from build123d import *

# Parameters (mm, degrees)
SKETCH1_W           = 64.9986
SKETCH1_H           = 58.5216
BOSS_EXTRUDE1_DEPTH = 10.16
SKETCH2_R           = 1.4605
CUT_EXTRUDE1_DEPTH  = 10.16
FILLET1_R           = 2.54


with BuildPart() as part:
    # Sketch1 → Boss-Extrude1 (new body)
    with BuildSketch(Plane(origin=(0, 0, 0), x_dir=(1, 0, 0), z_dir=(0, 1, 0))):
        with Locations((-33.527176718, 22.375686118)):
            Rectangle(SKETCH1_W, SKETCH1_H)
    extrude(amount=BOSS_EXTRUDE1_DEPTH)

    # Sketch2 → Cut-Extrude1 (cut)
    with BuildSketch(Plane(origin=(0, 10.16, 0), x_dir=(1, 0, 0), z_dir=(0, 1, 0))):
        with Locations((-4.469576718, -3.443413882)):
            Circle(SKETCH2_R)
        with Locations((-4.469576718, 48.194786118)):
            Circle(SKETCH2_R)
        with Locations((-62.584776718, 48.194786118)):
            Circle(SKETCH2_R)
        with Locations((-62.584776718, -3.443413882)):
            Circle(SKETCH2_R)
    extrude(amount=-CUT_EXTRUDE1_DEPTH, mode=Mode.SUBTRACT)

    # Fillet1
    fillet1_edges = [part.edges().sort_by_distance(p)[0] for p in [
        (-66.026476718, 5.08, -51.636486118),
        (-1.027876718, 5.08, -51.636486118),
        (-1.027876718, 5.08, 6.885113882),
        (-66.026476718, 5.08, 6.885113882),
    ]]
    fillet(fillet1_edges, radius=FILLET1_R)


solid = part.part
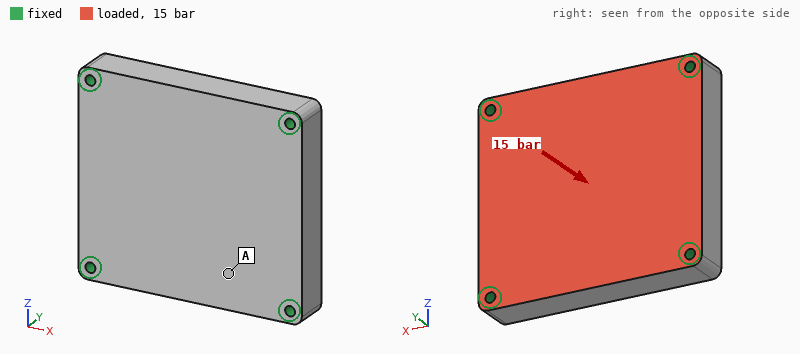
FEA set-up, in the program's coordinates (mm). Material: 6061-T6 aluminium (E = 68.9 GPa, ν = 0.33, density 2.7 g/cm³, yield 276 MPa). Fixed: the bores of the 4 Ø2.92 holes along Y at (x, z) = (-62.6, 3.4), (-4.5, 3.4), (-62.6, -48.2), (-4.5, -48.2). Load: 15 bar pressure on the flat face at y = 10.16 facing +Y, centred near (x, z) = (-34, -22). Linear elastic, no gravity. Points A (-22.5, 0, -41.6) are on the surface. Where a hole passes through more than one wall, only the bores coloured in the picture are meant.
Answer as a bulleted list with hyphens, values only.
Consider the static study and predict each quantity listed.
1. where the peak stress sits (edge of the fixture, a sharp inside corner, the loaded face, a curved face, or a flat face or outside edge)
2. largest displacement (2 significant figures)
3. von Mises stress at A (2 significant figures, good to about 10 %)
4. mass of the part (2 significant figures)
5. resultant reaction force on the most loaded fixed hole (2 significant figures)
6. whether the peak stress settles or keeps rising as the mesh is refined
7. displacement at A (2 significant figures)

- edge of the fixture
- 25 µm
- 13 MPa
- 100 g
- 1.4 kN
- keeps rising
- 18 µm
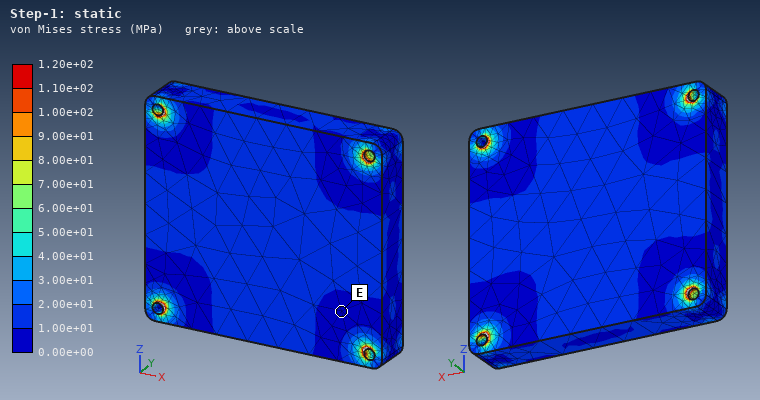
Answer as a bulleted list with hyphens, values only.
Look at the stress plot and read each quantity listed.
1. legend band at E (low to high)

- 0.00e+00 to 1.00e+01 MPa
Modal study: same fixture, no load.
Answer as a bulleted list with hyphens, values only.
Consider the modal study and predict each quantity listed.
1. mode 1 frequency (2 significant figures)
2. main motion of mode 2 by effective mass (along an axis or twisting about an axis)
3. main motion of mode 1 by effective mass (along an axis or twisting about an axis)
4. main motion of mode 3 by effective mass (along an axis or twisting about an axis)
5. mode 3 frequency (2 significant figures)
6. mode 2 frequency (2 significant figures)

- 8700 Hz
- twisting about X
- along Y
- twisting about Z
- 15 kHz
- 14 kHz
